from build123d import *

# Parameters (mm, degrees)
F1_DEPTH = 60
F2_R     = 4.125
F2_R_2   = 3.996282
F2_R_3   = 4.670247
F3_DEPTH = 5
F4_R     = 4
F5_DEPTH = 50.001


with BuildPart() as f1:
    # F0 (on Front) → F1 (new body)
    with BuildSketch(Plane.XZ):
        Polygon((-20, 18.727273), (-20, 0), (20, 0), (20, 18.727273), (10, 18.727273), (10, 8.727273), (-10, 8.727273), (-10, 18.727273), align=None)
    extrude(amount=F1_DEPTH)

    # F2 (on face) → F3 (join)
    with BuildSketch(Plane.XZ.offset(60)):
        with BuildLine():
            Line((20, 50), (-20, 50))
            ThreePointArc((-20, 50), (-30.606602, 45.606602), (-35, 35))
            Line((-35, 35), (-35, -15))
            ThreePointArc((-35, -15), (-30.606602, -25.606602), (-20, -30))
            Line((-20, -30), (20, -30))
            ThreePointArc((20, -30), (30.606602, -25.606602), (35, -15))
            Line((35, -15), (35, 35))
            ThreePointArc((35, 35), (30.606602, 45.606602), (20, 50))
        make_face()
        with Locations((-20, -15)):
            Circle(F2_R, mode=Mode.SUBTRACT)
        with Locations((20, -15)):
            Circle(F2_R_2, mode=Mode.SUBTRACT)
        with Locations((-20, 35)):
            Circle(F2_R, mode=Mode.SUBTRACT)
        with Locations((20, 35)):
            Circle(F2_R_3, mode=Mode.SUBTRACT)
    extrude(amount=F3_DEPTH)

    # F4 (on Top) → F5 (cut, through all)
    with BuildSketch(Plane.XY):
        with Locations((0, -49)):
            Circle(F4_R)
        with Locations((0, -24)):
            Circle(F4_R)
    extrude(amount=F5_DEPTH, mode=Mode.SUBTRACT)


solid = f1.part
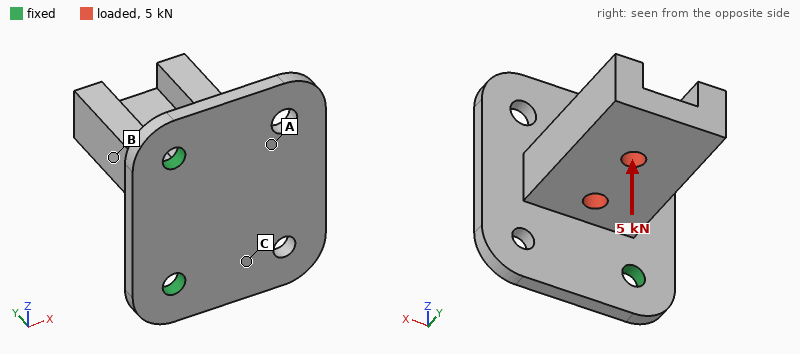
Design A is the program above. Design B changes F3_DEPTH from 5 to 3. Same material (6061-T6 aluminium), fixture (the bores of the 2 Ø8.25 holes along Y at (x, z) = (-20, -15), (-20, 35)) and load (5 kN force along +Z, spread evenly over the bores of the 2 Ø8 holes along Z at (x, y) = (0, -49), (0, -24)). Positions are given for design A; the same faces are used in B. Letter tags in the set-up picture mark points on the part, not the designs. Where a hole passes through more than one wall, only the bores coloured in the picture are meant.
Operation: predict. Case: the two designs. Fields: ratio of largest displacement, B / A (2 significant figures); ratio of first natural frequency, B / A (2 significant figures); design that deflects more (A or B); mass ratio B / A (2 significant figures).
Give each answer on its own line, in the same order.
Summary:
2.5
0.55
B
0.82
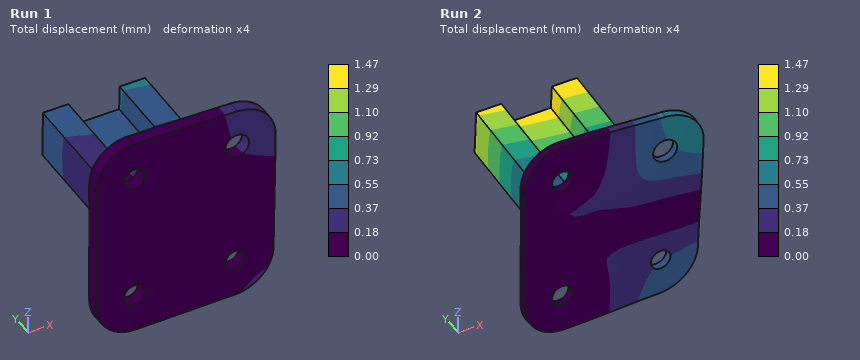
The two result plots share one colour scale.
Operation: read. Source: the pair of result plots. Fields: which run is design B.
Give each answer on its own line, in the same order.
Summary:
Run 2
